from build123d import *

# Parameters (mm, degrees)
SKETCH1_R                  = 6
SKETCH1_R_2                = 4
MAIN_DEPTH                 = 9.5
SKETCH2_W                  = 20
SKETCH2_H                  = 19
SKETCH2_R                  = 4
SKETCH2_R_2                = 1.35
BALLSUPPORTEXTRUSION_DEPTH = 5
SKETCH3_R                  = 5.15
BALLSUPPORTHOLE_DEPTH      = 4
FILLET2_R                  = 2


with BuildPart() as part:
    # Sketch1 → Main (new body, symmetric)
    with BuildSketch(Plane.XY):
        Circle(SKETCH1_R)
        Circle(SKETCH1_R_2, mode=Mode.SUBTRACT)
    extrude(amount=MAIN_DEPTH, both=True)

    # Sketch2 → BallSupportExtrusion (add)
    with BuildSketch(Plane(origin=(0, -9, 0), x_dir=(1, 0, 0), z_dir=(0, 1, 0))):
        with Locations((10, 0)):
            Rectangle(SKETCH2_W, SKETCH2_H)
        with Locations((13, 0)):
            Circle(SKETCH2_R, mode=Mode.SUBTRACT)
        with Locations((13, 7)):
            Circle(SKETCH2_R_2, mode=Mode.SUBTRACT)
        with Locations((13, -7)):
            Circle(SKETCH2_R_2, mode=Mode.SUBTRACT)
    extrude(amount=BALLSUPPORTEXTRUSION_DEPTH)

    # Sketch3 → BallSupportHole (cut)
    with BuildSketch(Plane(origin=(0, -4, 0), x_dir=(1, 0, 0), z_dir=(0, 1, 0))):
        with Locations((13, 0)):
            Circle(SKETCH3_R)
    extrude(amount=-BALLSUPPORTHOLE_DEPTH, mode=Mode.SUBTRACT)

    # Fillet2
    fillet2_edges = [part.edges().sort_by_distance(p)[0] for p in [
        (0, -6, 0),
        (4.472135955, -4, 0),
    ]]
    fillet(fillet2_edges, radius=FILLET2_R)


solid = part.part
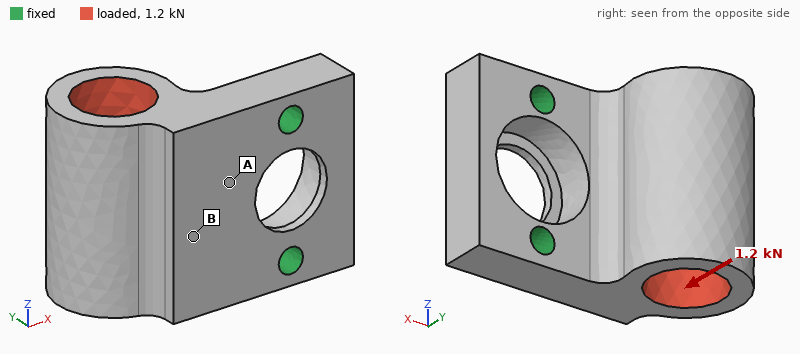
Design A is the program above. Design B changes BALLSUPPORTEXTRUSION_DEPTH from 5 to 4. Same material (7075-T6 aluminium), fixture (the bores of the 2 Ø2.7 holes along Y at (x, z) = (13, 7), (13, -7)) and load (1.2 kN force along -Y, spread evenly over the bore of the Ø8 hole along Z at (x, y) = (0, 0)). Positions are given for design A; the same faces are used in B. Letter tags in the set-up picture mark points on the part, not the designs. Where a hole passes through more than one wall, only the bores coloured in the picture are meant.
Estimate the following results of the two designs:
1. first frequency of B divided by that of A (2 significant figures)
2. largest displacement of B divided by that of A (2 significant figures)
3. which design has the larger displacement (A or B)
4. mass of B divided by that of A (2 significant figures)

0.74
1.8
B
0.93
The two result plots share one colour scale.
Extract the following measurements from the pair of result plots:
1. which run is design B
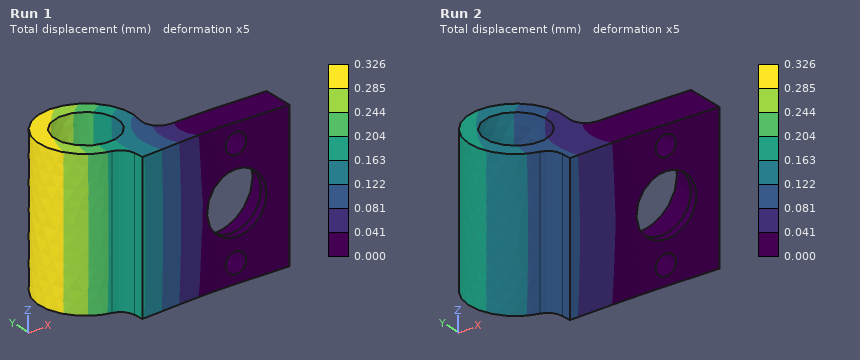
Run 1
